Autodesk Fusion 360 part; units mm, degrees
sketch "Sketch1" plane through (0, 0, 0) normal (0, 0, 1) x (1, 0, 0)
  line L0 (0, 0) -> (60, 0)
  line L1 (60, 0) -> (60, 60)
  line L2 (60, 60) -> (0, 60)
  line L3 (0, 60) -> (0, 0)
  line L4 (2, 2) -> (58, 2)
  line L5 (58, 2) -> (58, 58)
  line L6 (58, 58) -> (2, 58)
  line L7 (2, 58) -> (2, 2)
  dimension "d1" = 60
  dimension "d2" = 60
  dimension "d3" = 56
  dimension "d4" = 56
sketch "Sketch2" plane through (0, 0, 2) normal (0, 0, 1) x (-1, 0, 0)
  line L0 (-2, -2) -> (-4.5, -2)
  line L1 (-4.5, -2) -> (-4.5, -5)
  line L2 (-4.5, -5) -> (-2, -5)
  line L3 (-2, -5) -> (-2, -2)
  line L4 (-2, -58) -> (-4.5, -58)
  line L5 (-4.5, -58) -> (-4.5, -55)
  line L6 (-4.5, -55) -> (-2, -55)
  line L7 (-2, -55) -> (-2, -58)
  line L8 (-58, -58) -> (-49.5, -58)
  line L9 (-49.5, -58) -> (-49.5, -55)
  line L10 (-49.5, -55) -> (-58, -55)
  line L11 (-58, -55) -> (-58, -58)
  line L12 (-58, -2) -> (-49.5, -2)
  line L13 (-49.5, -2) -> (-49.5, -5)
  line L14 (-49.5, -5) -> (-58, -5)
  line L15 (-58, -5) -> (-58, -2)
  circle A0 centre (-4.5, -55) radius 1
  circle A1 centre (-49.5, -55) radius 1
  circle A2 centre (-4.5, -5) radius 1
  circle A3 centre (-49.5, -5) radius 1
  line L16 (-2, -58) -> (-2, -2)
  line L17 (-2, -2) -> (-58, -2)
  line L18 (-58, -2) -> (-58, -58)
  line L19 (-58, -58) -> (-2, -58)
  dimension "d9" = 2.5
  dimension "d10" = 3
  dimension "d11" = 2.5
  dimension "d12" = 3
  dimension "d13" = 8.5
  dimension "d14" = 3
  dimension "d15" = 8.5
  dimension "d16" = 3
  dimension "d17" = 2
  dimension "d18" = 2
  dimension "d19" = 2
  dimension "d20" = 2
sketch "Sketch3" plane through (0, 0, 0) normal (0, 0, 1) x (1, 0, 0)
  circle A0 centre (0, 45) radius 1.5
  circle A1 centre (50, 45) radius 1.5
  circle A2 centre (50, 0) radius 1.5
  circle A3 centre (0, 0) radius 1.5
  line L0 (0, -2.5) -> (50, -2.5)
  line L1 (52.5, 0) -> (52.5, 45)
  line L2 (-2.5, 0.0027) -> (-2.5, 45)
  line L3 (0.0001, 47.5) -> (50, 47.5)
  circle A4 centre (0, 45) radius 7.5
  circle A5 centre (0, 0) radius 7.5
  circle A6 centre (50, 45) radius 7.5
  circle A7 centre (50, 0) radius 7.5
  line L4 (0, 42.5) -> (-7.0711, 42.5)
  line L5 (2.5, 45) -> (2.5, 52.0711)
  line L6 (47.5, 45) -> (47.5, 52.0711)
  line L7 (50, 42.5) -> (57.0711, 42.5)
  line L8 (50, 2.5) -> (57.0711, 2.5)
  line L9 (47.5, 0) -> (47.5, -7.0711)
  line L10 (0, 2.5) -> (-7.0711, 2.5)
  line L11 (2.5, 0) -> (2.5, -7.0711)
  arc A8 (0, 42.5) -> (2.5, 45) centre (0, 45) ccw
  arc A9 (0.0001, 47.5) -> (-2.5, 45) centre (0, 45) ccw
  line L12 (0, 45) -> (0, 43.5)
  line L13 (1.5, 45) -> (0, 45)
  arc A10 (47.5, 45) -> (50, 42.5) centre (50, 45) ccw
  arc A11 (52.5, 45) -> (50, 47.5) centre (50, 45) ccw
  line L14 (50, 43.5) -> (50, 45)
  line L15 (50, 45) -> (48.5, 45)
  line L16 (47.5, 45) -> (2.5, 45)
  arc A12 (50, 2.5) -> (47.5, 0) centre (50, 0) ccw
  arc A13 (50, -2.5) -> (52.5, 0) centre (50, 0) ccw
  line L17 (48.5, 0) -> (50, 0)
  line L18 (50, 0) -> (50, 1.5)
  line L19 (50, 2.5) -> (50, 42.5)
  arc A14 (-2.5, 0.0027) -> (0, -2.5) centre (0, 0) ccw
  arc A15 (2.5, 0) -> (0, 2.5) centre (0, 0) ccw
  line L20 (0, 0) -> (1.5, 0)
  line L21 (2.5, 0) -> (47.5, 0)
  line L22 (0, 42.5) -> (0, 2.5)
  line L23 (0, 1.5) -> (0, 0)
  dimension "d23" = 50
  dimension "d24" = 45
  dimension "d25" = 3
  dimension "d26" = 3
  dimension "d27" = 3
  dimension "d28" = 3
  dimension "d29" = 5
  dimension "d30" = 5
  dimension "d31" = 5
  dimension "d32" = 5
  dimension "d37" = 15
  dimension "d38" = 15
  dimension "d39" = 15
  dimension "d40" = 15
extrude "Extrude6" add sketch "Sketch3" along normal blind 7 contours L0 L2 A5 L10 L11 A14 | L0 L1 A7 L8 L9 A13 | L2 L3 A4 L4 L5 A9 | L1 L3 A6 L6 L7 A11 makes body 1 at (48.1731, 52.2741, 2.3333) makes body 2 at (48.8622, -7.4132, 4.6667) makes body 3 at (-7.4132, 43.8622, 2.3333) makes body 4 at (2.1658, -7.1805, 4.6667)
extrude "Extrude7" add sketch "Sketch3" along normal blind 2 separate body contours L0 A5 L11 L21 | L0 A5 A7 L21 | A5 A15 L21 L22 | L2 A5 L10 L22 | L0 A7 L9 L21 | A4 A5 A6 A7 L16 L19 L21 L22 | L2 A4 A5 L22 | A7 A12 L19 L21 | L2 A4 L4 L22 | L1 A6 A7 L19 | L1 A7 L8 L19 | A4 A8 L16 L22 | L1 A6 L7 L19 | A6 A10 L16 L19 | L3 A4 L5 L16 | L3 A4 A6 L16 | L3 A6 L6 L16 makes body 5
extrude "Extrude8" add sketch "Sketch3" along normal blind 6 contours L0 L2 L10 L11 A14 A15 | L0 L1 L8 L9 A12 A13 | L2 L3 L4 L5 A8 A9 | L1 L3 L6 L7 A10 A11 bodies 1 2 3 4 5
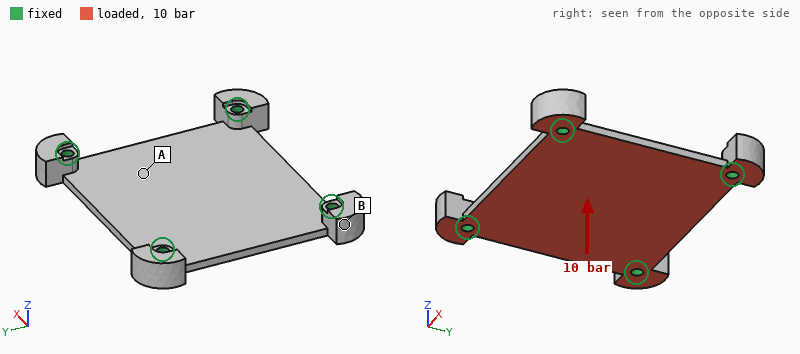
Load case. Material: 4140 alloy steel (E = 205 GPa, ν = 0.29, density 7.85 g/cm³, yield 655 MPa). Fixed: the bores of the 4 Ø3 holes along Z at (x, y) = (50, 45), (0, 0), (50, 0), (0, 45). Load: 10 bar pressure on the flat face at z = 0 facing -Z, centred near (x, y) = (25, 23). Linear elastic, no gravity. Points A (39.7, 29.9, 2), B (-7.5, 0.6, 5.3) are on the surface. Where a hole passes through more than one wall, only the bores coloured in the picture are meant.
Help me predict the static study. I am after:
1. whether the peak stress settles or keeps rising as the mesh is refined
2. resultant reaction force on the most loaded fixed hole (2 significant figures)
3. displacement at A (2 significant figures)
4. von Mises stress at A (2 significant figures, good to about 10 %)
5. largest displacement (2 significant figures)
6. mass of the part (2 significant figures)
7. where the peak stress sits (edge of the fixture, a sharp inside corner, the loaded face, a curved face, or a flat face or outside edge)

keeps rising
760 N
0.17 mm
120 MPa
0.25 mm
59 g
edge of the fixture
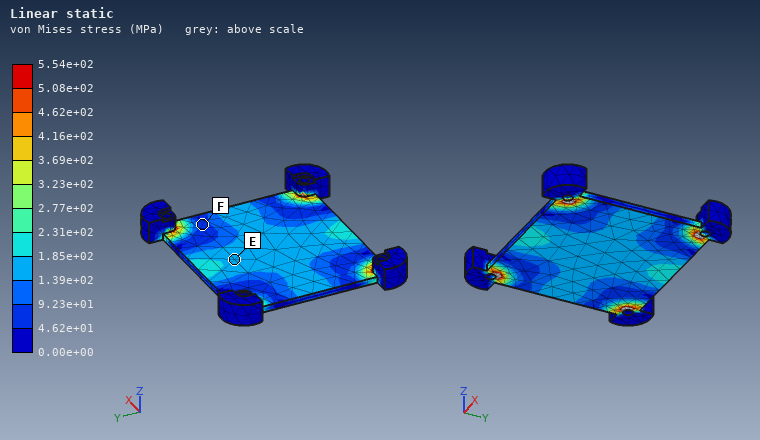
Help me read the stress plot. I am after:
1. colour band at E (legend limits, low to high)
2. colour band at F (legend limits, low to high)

1.39e+02 to 1.85e+02 MPa
4.62e+01 to 9.23e+01 MPa
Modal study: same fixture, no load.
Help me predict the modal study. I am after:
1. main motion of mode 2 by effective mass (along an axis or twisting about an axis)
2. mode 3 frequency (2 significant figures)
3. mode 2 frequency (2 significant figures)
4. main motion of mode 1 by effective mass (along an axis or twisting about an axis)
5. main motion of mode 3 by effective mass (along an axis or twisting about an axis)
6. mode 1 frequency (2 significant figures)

twisting about X
5900 Hz
5200 Hz
along Z
twisting about Y
3100 Hz
